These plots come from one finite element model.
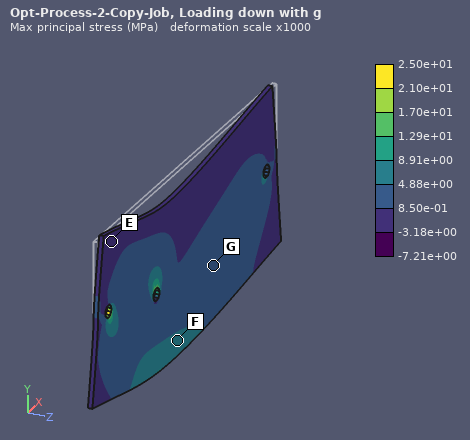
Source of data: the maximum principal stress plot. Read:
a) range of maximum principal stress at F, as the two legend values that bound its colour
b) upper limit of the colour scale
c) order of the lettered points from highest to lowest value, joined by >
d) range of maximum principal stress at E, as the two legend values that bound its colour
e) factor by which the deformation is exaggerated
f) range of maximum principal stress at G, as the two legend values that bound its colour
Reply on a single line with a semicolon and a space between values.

4.88e+00 to 8.91e+00 MPa; 2.50e+01 MPa; F > G > E; -3.18e+00 to 8.50e-01 MPa; 1000; 8.50e-01 to 4.88e+00 MPa
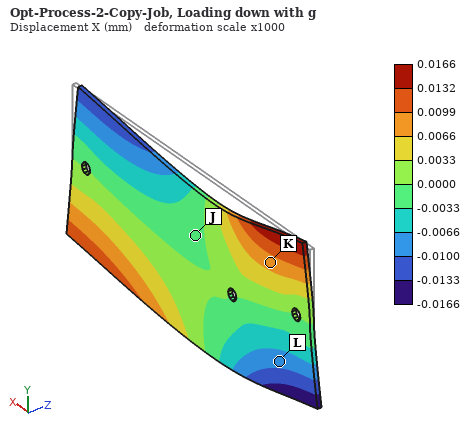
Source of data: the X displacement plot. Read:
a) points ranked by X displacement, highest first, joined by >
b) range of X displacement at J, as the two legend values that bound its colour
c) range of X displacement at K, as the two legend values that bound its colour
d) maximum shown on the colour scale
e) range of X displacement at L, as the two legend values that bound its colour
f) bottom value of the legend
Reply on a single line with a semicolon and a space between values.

K > J > L; -0.0033 to 0.0000 mm; 0.0066 to 0.0099 mm; 0.0166 mm; -0.0100 to -0.0066 mm; -0.0166 mm
